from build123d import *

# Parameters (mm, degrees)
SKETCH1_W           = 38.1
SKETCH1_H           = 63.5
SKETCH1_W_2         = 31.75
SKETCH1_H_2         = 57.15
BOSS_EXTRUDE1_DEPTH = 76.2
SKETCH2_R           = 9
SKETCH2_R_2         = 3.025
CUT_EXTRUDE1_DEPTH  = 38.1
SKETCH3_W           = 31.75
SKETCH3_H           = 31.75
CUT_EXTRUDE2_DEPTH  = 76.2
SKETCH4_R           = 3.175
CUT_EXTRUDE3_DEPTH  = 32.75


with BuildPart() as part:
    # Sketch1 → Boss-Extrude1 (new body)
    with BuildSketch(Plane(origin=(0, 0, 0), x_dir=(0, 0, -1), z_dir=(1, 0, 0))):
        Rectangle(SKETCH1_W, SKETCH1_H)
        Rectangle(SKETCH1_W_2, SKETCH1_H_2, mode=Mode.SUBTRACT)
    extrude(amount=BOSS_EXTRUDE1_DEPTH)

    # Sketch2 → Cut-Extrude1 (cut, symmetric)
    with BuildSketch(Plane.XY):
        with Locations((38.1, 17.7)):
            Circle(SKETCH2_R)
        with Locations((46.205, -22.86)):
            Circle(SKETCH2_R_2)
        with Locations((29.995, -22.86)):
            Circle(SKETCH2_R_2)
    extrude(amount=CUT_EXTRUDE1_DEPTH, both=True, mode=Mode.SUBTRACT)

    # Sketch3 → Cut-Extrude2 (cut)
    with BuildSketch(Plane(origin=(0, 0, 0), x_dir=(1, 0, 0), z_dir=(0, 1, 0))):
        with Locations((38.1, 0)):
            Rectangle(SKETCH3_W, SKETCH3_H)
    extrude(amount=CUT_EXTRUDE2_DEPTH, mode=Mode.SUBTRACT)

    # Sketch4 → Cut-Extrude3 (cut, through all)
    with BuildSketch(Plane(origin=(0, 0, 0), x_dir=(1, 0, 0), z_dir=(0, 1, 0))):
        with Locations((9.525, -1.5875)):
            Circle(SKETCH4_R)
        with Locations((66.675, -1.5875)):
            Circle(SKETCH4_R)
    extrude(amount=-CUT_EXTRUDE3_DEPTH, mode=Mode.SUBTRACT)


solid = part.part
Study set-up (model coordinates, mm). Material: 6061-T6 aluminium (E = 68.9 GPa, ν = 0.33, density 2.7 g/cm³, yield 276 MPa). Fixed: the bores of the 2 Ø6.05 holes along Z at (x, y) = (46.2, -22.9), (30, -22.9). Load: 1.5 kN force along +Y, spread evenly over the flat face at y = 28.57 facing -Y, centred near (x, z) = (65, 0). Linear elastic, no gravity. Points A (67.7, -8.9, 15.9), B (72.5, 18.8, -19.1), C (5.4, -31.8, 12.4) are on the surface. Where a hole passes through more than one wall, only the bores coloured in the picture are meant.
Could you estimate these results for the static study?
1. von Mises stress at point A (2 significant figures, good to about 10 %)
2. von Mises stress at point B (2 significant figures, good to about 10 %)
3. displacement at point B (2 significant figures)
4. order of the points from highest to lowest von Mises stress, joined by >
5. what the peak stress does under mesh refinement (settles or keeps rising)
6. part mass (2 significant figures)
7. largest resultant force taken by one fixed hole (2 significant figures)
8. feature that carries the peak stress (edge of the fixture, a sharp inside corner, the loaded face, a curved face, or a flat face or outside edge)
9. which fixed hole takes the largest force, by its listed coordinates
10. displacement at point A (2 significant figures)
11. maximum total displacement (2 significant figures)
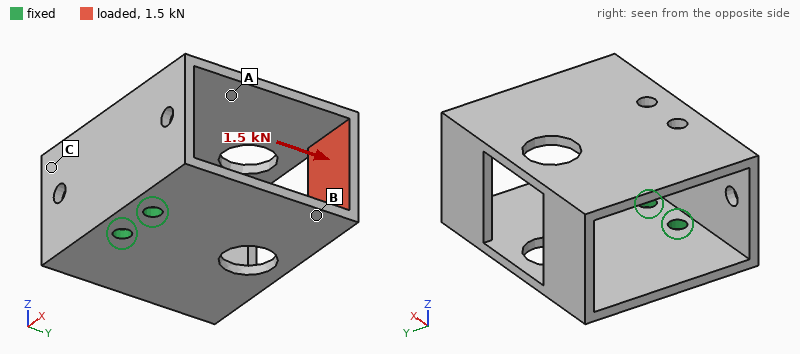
41 MPa
71 MPa
0.47 mm
B > A > C
keeps rising
110 g
2.6 kN
edge of the fixture
(46.2, -22.9)
0.86 mm
1.2 mm
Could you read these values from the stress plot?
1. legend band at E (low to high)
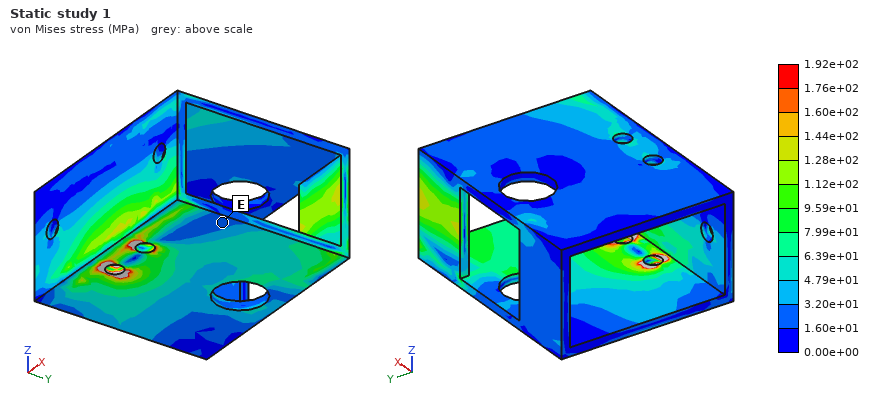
1.60e+01 to 3.20e+01 MPa
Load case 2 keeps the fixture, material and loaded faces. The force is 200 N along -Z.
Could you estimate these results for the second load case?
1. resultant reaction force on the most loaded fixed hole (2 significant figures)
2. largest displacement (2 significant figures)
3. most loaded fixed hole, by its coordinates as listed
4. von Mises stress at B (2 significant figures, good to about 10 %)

340 N
0.55 mm
(46.2, -22.9)
14 MPa
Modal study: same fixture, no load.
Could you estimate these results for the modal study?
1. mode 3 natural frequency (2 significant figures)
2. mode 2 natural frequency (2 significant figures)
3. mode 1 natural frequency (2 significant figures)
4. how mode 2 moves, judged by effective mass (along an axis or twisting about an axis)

1400 Hz
1000 Hz
490 Hz
along X
